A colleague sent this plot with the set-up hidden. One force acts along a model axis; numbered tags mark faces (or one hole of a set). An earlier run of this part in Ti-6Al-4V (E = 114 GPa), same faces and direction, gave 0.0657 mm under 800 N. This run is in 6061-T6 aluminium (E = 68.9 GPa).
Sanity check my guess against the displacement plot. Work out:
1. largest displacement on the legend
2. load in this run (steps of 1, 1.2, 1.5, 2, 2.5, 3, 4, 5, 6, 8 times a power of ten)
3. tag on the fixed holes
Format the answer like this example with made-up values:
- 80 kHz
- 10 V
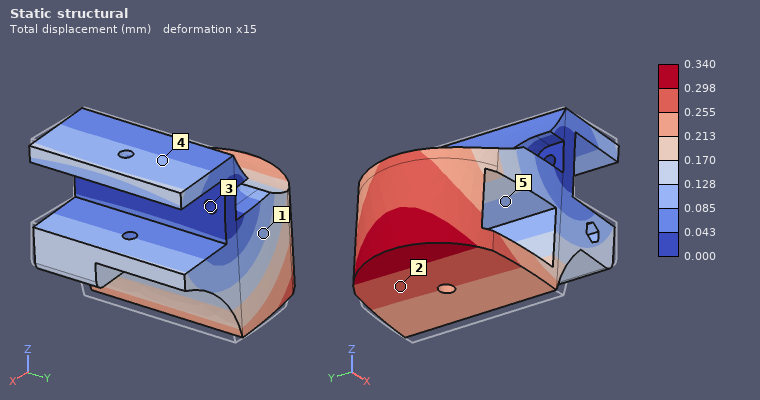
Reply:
- 0.340 mm
- 2.5 kN
- 3
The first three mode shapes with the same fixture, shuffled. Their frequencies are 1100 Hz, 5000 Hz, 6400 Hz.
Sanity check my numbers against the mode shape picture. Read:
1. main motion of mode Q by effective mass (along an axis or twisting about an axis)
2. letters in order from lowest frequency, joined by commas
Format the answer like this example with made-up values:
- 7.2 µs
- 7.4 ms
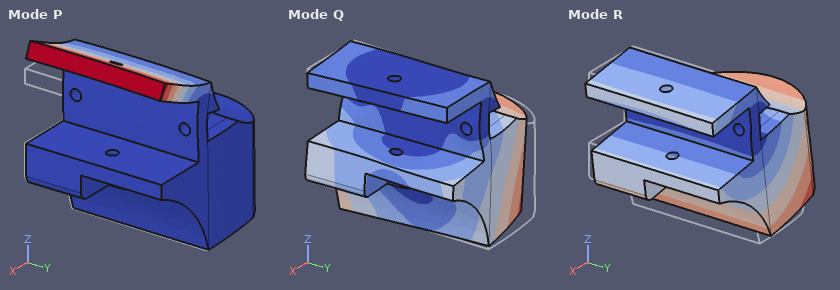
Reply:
- along Y
- R, Q, P
